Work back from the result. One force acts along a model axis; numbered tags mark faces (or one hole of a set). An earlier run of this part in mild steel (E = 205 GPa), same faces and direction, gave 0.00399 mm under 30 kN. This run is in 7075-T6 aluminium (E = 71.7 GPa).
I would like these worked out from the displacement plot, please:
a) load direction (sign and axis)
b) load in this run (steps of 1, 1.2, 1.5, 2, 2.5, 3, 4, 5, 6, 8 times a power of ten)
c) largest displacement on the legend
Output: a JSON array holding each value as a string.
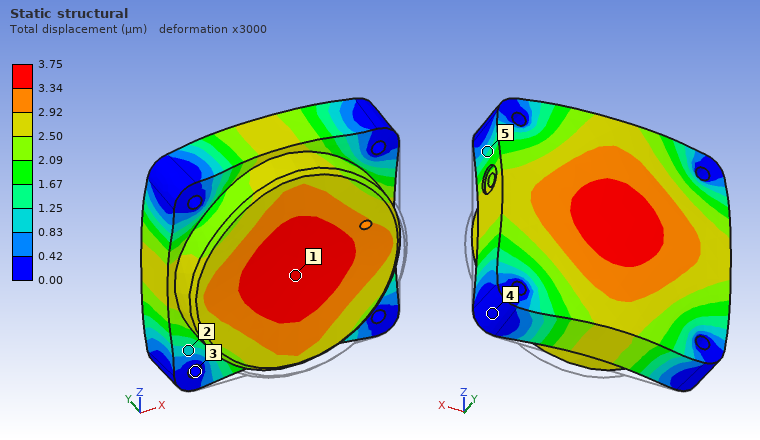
["+Y", "10 kN", "3.75 µm"]
